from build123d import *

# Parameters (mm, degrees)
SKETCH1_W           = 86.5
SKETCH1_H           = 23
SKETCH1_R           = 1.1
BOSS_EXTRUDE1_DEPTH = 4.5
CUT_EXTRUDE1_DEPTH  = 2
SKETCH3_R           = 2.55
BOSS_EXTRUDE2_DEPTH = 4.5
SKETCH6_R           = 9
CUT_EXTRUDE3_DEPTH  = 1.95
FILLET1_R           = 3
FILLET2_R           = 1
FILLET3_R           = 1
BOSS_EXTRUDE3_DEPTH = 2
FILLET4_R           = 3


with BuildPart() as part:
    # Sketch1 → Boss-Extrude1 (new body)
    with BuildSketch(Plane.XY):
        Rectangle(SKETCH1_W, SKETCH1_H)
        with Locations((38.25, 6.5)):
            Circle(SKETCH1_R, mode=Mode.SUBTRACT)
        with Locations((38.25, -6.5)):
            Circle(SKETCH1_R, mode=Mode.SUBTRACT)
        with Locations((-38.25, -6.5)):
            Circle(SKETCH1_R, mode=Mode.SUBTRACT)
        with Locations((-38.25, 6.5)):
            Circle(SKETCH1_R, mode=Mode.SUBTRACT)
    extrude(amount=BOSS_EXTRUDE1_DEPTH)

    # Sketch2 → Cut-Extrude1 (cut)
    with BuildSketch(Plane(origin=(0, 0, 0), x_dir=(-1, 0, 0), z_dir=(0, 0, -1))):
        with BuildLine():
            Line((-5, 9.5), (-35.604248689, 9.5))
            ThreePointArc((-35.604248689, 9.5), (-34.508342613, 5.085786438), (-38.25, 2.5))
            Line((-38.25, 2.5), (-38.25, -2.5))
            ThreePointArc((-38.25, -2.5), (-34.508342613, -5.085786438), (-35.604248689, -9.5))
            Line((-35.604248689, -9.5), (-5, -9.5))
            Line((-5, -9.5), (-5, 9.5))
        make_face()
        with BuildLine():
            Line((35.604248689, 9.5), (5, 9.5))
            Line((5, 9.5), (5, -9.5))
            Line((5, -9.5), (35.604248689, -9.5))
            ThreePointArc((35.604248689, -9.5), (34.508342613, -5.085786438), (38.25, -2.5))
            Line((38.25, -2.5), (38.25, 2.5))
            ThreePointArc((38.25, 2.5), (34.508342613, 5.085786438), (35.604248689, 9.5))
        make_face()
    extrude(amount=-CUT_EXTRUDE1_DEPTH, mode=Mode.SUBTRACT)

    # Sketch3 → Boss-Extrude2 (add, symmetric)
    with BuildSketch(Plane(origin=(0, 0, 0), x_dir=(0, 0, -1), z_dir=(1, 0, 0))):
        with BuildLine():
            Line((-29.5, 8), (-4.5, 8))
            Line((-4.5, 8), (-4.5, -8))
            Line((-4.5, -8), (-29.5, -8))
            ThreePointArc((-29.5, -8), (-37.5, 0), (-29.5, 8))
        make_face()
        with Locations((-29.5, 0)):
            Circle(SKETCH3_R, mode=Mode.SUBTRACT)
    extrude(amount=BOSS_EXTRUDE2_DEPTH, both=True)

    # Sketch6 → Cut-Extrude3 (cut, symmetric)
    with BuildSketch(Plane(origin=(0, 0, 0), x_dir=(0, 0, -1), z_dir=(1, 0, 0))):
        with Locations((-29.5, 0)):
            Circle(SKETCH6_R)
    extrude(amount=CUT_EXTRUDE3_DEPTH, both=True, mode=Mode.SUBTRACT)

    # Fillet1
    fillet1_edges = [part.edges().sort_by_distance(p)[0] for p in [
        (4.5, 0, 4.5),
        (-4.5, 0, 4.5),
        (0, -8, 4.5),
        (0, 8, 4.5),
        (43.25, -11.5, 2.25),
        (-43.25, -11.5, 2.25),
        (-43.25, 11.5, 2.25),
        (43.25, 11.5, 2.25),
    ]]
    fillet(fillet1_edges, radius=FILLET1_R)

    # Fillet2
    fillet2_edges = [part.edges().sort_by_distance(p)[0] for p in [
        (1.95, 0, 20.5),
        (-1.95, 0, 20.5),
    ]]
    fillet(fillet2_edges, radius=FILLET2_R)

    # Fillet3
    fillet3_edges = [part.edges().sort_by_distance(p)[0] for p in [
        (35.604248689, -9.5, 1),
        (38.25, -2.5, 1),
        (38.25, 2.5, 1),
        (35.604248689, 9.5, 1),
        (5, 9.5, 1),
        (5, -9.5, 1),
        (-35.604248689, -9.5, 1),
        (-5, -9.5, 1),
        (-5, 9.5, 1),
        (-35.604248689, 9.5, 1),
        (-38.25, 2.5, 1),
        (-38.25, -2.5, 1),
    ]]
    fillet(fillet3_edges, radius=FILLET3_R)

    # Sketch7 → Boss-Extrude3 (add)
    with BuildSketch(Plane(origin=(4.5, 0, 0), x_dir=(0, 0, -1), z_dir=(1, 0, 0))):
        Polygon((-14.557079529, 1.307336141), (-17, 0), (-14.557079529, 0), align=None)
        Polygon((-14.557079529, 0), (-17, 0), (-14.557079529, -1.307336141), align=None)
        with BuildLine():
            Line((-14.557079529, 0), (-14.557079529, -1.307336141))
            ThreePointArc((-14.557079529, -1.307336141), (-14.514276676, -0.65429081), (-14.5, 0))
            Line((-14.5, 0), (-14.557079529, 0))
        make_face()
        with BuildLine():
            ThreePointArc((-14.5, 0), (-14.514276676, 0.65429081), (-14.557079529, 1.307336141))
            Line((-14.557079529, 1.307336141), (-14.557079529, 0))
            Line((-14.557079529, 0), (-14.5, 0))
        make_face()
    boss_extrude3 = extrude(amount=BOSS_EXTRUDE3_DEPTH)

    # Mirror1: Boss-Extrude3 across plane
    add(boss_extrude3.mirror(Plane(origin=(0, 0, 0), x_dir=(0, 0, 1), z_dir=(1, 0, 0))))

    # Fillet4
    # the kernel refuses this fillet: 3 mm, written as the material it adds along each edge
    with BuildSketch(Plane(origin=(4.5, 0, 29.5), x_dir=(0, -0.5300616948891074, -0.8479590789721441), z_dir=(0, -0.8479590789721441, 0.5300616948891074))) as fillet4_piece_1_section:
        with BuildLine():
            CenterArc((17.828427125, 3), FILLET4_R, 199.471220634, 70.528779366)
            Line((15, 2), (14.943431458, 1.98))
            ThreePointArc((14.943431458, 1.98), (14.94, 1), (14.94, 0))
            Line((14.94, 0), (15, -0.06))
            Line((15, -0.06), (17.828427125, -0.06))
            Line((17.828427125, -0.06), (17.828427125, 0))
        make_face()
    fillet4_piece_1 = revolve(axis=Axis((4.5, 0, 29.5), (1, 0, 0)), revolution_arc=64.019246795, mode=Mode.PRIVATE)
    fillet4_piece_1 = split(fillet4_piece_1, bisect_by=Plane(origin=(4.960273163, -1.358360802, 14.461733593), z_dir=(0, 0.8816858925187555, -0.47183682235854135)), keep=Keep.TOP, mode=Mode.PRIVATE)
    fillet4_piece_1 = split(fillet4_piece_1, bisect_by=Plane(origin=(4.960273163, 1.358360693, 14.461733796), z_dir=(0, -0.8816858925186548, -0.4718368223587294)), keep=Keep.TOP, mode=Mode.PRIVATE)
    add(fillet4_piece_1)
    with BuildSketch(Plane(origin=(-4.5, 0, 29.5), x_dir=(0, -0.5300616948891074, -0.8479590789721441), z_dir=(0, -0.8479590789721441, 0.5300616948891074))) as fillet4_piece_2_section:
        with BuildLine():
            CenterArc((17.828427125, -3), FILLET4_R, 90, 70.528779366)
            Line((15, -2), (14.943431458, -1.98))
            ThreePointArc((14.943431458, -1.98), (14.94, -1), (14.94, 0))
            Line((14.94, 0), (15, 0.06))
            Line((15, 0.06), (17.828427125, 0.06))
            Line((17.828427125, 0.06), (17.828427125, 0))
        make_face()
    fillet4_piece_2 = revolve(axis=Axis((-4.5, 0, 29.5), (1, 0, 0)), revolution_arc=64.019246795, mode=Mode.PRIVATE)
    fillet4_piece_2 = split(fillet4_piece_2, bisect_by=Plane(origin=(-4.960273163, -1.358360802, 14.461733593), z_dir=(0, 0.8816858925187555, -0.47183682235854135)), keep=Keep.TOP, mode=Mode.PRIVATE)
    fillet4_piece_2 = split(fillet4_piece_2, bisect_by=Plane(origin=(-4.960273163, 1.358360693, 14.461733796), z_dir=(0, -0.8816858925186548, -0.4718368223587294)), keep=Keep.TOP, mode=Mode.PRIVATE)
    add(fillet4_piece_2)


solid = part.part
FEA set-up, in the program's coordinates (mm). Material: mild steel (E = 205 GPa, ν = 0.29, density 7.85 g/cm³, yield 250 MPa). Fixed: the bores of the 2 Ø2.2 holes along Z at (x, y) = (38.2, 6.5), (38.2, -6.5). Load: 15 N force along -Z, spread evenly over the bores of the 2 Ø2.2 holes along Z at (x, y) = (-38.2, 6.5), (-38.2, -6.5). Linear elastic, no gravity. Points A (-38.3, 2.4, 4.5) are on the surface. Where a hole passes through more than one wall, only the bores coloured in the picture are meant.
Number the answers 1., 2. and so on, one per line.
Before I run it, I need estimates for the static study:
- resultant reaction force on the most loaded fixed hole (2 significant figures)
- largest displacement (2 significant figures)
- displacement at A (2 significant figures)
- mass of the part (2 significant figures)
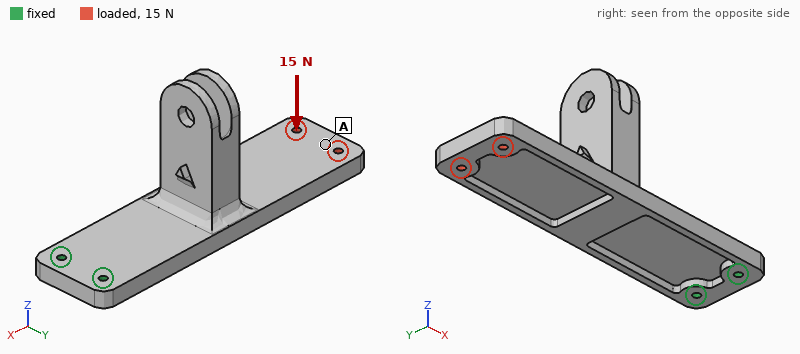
1. 20 N
2. 0.15 mm
3. 0.14 mm
4. 80 g
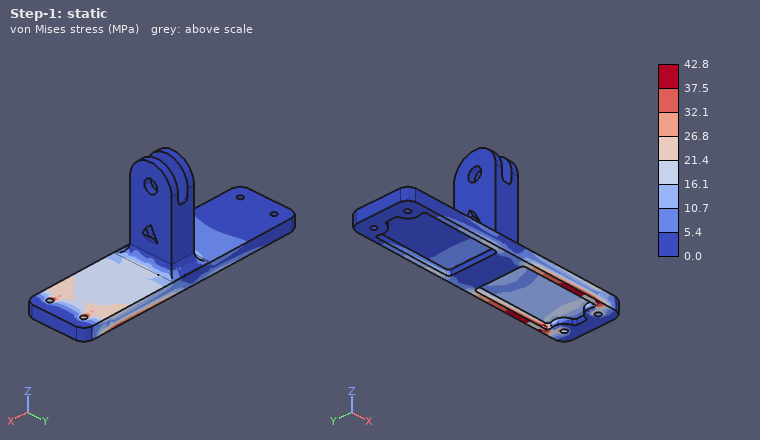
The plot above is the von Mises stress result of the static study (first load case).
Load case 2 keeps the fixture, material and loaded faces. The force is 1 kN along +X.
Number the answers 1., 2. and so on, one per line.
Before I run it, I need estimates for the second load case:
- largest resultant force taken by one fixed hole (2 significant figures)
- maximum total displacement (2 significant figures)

1. 500 N
2. 0.15 mm
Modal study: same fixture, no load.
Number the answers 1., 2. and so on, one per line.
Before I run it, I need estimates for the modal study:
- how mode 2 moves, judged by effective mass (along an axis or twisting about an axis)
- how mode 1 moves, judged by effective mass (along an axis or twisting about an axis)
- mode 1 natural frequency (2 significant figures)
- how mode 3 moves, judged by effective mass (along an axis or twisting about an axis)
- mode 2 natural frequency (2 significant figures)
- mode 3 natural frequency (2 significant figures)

1. along Y
2. along Z
3. 360 Hz
4. along Z
5. 1200 Hz
6. 2000 Hz
